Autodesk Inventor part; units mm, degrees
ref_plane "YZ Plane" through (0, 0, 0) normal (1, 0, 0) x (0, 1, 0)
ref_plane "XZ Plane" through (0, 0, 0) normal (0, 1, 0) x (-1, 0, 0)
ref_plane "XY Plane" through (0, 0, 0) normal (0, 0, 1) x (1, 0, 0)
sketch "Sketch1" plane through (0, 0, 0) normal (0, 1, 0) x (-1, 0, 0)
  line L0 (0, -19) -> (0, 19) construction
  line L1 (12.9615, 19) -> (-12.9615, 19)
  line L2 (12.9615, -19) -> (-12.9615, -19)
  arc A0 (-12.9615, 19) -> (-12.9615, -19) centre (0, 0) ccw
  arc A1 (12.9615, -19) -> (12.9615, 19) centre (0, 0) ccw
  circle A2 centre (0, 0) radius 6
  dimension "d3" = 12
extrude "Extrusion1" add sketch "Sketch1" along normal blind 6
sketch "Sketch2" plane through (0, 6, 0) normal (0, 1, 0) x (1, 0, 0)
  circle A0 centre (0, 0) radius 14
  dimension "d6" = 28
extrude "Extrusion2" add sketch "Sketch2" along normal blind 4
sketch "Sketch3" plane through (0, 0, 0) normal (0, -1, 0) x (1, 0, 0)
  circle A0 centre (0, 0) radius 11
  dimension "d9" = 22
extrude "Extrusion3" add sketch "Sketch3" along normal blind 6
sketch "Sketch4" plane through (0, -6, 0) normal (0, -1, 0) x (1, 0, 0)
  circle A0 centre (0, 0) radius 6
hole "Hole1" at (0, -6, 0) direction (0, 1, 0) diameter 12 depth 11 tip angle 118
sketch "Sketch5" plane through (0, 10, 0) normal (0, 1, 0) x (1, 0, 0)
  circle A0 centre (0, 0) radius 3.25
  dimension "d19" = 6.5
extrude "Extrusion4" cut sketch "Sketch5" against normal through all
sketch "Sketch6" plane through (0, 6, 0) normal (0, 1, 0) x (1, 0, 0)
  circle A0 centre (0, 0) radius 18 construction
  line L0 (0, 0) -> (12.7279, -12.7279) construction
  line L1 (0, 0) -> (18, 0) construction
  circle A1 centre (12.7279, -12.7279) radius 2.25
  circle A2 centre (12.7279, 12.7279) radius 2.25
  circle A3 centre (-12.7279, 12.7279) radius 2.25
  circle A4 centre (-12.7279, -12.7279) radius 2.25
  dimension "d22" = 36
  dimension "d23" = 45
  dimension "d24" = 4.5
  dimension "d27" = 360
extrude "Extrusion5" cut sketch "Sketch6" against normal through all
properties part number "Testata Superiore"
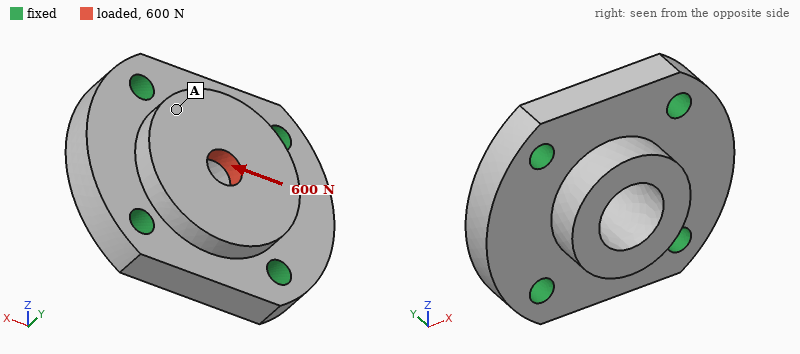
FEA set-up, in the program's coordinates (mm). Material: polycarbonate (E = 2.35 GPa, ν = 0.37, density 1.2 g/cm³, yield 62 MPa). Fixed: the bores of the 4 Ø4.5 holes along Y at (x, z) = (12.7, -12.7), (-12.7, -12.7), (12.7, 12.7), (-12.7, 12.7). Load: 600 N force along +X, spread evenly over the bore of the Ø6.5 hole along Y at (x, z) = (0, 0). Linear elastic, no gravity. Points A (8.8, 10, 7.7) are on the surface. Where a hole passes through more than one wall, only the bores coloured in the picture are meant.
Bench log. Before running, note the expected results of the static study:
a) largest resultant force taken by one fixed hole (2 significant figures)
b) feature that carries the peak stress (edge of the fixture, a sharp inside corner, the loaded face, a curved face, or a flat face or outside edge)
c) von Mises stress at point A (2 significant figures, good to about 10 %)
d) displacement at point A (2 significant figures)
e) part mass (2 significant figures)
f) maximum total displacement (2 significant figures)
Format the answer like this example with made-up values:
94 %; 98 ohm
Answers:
170 N; the loaded face; 2.2 MPa; 17 µm; 14 g; 43 µm
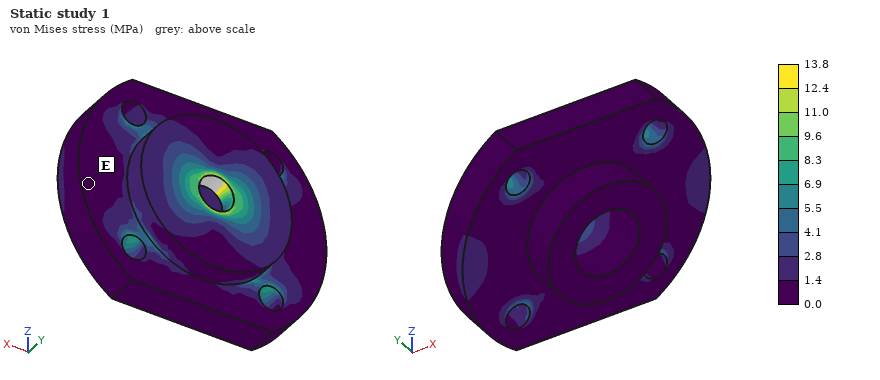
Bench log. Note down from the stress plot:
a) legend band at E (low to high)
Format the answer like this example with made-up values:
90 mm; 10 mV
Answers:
0.0 to 1.4 MPa
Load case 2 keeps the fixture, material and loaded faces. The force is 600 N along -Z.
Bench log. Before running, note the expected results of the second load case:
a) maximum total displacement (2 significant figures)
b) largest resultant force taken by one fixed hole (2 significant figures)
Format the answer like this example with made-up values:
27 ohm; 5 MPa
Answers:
44 µm; 170 N
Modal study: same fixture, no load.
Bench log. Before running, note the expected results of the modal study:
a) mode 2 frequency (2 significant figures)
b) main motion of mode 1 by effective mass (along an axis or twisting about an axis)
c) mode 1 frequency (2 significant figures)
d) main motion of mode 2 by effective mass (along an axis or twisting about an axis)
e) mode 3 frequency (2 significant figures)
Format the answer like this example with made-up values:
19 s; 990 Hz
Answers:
9100 Hz; along Y; 8500 Hz; twisting about Z; 10 kHz
